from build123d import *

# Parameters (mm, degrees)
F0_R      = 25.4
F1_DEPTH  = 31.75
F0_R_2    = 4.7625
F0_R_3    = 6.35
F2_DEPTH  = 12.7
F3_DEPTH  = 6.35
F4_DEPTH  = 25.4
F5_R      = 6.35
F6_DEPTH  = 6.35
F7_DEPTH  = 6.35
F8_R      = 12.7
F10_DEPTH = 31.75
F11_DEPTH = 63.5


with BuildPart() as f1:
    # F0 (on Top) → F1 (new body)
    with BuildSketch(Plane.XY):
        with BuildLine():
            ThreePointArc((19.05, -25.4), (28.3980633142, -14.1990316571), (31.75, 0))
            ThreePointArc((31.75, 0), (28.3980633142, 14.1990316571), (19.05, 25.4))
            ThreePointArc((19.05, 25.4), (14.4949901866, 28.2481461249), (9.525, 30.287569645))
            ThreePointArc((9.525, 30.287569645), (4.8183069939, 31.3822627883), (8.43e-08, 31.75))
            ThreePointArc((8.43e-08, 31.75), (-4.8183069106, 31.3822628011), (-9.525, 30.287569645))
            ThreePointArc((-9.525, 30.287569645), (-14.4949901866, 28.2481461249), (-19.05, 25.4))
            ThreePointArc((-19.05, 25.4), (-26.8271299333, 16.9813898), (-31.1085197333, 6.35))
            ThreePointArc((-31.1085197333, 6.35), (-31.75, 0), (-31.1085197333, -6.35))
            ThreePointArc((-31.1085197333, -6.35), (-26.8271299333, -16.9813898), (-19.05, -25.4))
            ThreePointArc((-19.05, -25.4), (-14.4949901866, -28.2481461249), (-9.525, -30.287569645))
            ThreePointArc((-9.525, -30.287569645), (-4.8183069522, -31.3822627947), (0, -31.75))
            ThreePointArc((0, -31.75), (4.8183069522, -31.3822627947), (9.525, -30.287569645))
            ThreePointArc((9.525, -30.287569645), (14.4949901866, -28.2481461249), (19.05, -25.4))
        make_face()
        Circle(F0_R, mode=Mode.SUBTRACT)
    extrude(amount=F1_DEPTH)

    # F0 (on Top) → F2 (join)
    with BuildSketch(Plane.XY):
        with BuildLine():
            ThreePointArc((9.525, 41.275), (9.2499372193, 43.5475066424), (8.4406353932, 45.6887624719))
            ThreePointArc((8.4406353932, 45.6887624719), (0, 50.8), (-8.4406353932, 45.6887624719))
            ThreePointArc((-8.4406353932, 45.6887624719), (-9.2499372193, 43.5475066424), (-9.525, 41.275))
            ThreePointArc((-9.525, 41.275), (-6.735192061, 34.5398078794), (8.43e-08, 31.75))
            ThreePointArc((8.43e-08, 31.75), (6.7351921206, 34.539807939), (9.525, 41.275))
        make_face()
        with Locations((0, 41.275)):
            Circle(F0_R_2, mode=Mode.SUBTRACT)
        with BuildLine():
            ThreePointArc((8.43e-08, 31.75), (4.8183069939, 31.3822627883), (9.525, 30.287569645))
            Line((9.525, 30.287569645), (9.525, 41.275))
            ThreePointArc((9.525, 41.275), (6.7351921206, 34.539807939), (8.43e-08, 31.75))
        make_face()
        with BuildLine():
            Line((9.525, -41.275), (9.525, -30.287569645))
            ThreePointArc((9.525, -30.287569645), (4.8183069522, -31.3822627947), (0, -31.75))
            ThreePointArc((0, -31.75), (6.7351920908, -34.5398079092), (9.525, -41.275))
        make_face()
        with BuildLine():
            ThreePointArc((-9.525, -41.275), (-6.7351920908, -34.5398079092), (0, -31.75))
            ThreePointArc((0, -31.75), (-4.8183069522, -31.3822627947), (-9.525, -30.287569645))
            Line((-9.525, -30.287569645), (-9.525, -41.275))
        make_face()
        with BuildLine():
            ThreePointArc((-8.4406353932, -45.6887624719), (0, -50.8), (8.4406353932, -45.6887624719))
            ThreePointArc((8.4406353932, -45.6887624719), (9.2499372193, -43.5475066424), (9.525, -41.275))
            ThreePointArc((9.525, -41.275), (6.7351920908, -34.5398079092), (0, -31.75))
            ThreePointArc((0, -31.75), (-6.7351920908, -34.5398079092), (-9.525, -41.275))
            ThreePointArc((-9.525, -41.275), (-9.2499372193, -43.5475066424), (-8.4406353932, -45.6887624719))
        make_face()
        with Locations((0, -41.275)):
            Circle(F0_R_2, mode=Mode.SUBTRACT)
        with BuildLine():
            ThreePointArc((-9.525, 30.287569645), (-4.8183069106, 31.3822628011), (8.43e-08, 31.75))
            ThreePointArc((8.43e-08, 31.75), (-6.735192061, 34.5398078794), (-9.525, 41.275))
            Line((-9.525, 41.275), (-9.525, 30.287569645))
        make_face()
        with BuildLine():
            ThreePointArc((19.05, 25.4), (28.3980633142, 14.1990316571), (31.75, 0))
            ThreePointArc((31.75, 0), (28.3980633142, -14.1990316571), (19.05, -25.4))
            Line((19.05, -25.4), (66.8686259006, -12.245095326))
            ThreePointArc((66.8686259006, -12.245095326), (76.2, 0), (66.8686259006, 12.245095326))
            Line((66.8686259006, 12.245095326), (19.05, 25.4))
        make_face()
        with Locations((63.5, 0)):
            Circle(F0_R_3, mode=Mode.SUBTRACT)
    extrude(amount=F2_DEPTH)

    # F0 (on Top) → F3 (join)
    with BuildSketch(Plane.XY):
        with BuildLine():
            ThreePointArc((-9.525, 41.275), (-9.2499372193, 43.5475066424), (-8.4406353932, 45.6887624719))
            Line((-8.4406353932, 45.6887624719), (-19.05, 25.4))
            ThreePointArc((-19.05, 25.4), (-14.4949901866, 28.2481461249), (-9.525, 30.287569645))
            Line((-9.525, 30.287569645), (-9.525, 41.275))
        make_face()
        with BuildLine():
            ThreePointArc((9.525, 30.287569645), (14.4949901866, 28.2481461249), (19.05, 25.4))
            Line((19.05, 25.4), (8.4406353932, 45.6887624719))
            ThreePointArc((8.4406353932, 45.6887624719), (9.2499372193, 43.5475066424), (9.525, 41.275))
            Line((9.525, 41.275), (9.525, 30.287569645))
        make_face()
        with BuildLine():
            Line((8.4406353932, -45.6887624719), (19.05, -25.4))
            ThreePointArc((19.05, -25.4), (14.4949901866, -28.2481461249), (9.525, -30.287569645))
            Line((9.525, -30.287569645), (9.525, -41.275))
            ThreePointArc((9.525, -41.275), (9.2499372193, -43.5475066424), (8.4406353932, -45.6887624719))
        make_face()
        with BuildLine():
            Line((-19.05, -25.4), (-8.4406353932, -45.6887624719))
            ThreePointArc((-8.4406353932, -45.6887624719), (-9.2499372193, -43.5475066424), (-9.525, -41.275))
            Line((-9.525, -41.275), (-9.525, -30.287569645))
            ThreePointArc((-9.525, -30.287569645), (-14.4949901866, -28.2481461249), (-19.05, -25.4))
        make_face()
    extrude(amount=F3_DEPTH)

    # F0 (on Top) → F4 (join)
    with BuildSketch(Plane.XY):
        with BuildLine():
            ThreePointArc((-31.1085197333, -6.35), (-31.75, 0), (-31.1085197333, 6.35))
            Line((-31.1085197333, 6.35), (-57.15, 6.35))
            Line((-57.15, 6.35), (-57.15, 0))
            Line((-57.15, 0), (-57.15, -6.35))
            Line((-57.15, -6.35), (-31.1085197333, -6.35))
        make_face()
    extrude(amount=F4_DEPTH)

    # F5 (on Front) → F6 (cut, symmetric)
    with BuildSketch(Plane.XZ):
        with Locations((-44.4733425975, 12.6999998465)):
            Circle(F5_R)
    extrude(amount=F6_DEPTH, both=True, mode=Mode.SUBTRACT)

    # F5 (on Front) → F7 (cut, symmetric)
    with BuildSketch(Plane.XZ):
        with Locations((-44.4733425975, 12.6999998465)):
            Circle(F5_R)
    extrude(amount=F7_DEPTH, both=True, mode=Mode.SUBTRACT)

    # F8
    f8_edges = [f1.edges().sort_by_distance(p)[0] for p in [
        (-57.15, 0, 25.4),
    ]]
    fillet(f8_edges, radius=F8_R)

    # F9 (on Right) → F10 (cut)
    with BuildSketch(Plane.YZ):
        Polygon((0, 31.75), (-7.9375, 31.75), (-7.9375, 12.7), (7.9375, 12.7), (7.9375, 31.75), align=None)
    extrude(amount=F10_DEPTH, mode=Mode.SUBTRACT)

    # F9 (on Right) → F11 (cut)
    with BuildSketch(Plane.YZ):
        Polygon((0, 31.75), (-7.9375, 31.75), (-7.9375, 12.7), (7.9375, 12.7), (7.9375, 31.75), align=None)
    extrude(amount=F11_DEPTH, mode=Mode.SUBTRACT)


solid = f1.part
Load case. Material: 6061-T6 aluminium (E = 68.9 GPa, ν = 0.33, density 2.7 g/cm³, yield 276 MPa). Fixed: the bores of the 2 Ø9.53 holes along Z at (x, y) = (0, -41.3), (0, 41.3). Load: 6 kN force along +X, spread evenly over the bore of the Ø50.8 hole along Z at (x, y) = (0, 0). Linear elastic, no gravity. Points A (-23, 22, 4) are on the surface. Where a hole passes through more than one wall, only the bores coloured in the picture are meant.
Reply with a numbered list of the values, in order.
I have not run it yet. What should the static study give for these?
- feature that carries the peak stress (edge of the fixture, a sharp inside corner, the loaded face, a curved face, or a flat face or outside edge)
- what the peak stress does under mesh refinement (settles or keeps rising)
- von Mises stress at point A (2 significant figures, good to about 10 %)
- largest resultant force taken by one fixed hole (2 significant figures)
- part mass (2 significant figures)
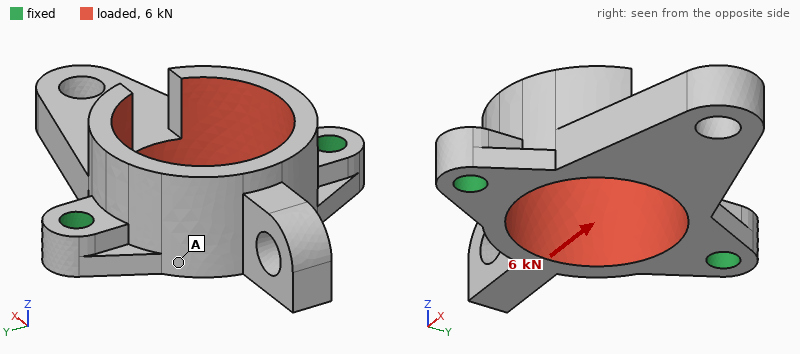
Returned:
1. edge of the fixture
2. keeps rising
3. 11 MPa
4. 3.0 kN
5. 180 g
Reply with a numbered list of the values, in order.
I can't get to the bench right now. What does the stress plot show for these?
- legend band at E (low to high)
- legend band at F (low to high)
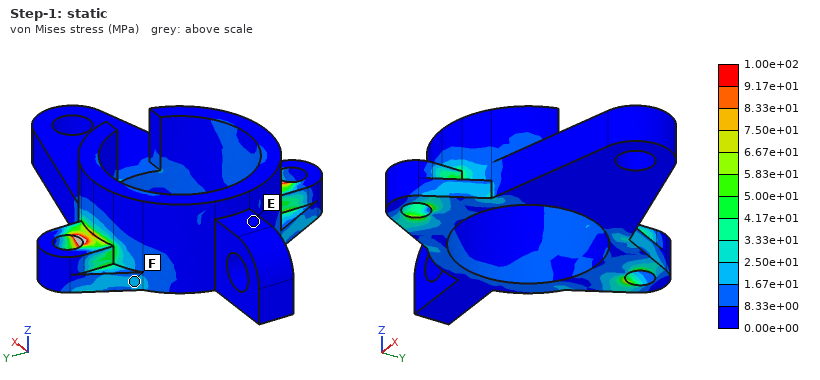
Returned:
1. 0.00e+00 to 8.33e+00 MPa
2. 1.67e+01 to 2.50e+01 MPa
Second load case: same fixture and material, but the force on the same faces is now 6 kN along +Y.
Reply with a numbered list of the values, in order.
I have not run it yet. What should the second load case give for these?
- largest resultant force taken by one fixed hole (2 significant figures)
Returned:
1. 3.1 kN
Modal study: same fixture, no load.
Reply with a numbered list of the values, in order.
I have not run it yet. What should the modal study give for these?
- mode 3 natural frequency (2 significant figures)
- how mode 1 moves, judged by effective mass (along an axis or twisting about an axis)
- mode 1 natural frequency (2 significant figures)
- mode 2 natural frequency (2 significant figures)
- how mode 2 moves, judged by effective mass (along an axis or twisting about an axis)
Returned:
1. 6500 Hz
2. along Z
3. 1900 Hz
4. 3300 Hz
5. along Z
